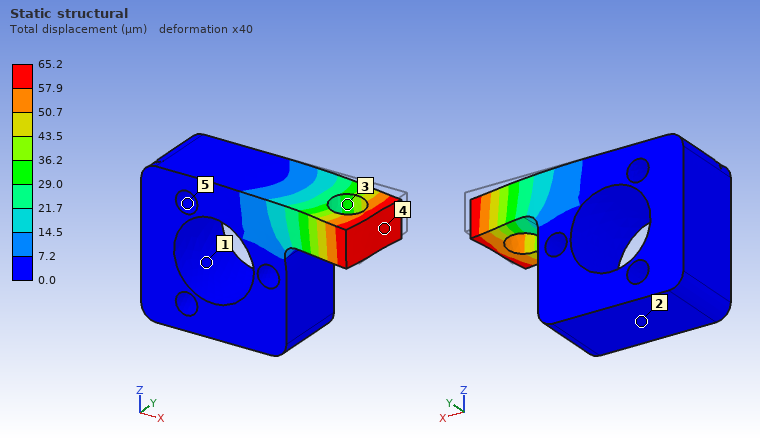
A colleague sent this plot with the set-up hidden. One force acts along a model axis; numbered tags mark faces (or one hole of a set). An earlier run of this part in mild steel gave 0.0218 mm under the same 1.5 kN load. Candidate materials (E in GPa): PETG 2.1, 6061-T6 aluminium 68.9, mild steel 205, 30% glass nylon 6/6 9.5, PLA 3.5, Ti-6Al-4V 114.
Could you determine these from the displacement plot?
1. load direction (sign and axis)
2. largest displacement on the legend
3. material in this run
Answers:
-Y
65.2 µm
6061-T6 aluminium
